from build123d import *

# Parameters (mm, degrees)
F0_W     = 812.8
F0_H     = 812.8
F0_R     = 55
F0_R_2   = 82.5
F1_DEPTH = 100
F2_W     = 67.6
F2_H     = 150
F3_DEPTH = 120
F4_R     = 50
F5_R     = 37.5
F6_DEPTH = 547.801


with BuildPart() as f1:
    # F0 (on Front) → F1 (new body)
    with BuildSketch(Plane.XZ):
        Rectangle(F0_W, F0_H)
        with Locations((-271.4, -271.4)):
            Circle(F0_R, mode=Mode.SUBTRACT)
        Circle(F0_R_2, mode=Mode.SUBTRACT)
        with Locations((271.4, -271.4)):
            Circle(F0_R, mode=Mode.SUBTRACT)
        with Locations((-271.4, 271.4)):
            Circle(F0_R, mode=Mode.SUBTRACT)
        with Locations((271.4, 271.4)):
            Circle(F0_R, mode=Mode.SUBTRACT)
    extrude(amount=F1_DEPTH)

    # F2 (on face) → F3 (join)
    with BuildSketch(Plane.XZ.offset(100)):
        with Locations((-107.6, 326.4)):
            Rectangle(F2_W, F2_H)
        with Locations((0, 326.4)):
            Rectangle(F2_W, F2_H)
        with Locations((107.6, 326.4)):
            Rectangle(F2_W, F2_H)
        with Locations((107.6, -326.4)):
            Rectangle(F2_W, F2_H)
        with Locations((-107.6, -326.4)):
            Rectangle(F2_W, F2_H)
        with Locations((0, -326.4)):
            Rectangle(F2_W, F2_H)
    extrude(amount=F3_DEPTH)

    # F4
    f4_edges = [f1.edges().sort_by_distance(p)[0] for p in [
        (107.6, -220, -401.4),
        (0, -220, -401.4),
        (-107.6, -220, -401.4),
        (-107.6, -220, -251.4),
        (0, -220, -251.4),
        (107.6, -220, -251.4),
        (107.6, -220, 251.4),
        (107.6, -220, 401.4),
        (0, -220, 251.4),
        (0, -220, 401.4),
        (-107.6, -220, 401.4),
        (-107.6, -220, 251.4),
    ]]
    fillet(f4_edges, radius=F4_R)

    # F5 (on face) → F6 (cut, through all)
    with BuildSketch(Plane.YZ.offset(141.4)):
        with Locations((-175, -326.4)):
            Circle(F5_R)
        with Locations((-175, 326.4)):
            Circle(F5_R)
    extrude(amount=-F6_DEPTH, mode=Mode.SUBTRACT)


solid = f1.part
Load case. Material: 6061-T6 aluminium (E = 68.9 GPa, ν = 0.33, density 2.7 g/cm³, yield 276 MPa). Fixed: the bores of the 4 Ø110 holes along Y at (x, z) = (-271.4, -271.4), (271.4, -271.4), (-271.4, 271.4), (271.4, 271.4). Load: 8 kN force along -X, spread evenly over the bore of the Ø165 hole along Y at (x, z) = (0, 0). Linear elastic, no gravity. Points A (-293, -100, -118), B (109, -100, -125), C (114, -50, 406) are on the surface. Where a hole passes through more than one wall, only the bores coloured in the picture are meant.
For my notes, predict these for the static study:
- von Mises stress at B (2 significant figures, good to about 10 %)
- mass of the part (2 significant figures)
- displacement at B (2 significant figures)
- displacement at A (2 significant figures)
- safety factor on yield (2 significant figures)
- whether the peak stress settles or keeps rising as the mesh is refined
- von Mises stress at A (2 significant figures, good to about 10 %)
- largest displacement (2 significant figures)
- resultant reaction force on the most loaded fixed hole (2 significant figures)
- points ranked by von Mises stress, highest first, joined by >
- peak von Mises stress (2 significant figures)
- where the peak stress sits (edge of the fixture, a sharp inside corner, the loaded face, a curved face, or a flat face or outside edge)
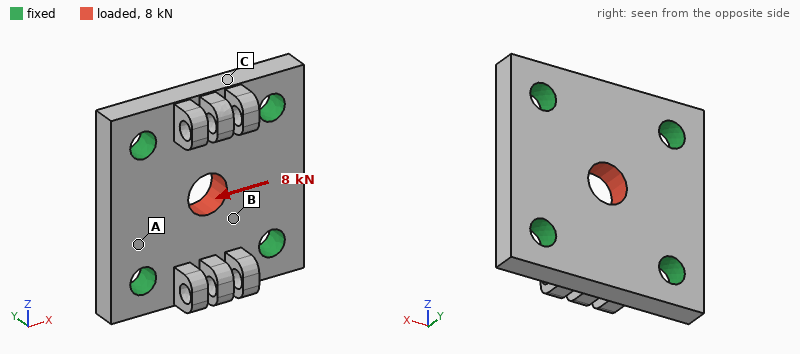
0.12 MPa
180 kg
0.33 µm
0.26 µm
1000
settles
0.066 MPa
0.62 µm
2.2 kN
B > A > C
0.27 MPa
the loaded face
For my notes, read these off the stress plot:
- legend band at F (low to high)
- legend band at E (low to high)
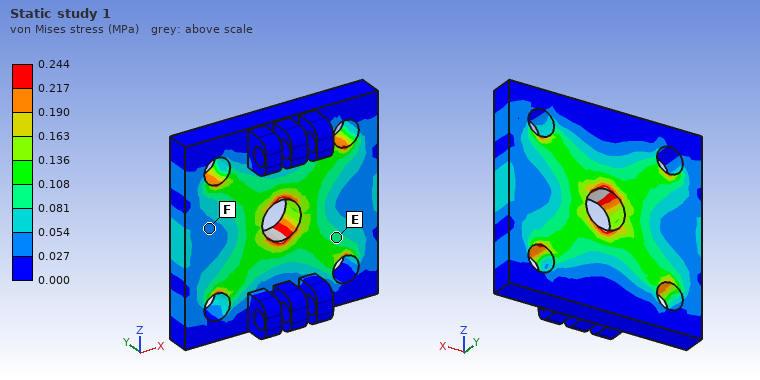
0.027 to 0.054 MPa
0.081 to 0.108 MPa
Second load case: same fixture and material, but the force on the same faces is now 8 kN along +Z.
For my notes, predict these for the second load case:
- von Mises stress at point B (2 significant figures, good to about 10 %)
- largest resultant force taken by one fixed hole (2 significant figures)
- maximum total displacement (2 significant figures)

0.12 MPa
2.2 kN
0.62 µm
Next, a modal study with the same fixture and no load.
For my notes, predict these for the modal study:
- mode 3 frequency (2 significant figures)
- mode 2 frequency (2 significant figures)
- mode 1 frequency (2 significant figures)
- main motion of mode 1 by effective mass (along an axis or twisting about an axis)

1500 Hz
1500 Hz
1300 Hz
along Y
